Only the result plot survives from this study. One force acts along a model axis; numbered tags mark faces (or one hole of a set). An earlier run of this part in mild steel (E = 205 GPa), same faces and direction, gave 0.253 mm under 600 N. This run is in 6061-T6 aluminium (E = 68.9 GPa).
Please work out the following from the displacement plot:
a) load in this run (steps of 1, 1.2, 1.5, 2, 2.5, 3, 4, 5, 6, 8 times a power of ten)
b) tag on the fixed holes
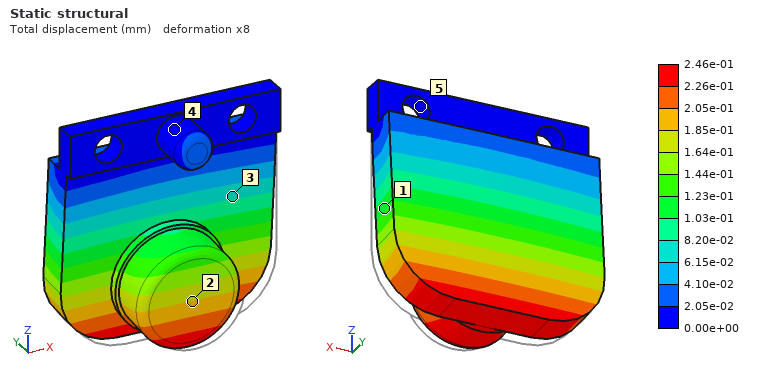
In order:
200 N
5
